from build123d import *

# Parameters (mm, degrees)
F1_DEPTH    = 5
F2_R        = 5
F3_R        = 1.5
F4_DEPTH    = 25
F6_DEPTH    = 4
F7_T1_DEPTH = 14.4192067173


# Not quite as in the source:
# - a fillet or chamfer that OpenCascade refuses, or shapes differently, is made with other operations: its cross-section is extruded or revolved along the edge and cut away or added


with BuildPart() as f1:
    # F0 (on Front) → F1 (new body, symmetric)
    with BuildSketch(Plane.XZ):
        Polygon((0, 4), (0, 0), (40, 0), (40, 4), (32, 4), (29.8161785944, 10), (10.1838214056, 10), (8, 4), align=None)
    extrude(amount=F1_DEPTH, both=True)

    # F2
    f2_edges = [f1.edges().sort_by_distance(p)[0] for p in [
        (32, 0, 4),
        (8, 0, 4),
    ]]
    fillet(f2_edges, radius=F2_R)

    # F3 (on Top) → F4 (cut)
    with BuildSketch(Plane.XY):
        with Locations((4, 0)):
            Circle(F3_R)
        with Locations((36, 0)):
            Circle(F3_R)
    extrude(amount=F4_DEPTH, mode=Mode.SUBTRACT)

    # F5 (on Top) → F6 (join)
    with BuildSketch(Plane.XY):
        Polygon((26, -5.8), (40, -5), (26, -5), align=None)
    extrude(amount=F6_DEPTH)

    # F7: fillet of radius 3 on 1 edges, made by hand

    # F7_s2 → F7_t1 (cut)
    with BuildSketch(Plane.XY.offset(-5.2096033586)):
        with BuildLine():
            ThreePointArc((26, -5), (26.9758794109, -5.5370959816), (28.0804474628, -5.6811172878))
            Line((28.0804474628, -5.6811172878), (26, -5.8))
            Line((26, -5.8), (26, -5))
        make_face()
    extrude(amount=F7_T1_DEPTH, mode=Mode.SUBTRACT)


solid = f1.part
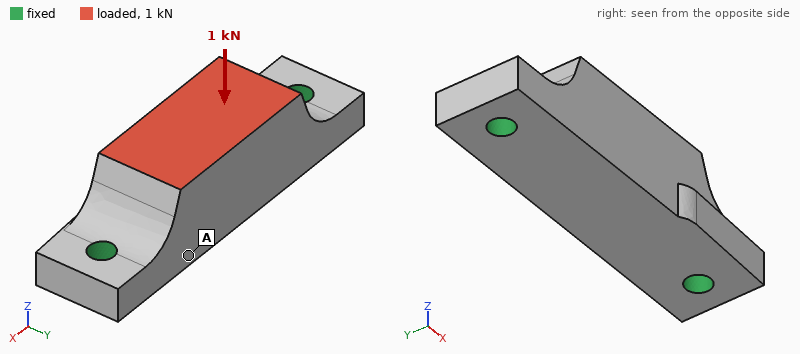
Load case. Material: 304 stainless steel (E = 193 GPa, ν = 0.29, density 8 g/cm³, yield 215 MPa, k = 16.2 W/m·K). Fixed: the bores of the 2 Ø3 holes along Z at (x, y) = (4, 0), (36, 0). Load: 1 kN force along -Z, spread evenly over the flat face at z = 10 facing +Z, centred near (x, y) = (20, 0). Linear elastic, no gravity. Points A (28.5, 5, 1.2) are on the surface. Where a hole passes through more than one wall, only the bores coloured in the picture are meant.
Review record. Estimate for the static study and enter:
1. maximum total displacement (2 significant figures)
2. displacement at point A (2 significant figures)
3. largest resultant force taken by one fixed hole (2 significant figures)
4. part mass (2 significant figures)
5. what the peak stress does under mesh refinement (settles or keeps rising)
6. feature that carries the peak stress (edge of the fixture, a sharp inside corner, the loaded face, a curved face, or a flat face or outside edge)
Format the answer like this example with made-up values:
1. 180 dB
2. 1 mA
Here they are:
1. 3.0 µm
2. 2.1 µm
3. 620 N
4. 23 g
5. keeps rising
6. edge of the fixture
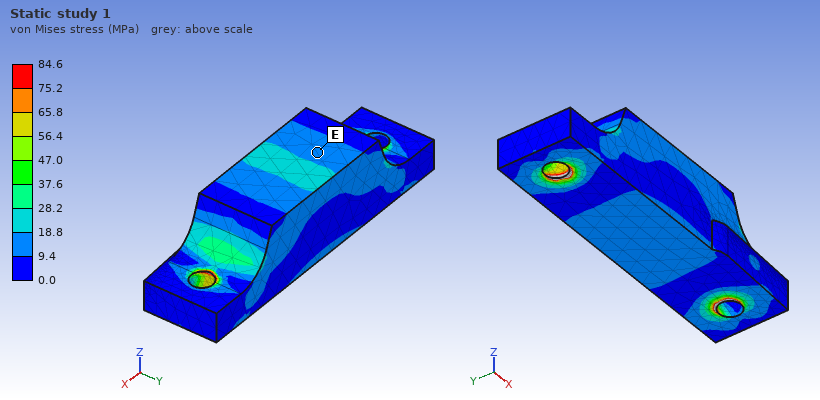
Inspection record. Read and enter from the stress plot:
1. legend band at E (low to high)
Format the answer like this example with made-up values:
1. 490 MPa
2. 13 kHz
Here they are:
1. 9.4 to 18.8 MPa
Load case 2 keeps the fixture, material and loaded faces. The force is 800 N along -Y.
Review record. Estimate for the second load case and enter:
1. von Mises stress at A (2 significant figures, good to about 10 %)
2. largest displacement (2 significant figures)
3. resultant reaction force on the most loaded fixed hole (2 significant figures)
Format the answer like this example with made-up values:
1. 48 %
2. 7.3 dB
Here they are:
1. 21 MPa
2. 12 µm
3. 400 N
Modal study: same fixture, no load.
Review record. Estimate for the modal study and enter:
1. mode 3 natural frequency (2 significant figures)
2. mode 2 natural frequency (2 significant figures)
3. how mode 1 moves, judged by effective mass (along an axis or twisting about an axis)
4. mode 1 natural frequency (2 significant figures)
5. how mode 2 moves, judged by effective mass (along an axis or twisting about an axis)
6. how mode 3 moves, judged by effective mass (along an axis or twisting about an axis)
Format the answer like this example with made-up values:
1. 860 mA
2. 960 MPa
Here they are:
1. 30 kHz
2. 24 kHz
3. along Y
4. 17 kHz
5. along Z
6. along Y
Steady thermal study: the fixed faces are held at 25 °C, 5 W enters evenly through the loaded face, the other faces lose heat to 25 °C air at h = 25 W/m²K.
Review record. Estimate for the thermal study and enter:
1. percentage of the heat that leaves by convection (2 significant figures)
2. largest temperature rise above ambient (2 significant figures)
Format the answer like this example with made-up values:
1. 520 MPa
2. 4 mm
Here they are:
1. 10 %
2. 33 K
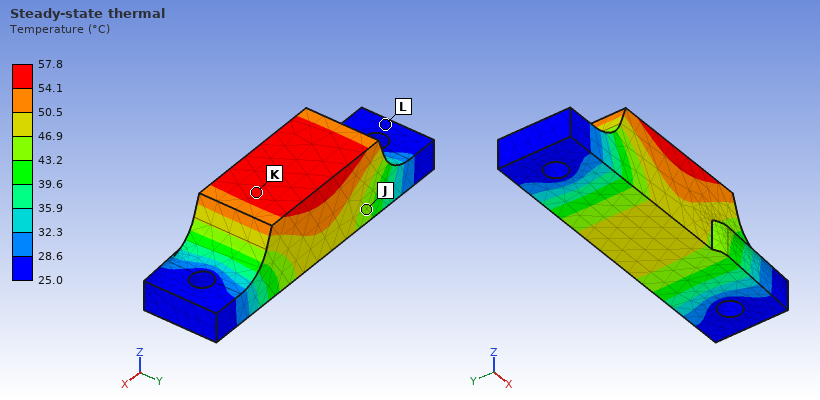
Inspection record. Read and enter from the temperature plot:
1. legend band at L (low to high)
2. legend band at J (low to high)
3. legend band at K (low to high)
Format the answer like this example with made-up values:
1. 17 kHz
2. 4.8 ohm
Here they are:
1. 25.0 to 28.6 °C
2. 43.2 to 46.9 °C
3. 54.1 to 57.8 °C
